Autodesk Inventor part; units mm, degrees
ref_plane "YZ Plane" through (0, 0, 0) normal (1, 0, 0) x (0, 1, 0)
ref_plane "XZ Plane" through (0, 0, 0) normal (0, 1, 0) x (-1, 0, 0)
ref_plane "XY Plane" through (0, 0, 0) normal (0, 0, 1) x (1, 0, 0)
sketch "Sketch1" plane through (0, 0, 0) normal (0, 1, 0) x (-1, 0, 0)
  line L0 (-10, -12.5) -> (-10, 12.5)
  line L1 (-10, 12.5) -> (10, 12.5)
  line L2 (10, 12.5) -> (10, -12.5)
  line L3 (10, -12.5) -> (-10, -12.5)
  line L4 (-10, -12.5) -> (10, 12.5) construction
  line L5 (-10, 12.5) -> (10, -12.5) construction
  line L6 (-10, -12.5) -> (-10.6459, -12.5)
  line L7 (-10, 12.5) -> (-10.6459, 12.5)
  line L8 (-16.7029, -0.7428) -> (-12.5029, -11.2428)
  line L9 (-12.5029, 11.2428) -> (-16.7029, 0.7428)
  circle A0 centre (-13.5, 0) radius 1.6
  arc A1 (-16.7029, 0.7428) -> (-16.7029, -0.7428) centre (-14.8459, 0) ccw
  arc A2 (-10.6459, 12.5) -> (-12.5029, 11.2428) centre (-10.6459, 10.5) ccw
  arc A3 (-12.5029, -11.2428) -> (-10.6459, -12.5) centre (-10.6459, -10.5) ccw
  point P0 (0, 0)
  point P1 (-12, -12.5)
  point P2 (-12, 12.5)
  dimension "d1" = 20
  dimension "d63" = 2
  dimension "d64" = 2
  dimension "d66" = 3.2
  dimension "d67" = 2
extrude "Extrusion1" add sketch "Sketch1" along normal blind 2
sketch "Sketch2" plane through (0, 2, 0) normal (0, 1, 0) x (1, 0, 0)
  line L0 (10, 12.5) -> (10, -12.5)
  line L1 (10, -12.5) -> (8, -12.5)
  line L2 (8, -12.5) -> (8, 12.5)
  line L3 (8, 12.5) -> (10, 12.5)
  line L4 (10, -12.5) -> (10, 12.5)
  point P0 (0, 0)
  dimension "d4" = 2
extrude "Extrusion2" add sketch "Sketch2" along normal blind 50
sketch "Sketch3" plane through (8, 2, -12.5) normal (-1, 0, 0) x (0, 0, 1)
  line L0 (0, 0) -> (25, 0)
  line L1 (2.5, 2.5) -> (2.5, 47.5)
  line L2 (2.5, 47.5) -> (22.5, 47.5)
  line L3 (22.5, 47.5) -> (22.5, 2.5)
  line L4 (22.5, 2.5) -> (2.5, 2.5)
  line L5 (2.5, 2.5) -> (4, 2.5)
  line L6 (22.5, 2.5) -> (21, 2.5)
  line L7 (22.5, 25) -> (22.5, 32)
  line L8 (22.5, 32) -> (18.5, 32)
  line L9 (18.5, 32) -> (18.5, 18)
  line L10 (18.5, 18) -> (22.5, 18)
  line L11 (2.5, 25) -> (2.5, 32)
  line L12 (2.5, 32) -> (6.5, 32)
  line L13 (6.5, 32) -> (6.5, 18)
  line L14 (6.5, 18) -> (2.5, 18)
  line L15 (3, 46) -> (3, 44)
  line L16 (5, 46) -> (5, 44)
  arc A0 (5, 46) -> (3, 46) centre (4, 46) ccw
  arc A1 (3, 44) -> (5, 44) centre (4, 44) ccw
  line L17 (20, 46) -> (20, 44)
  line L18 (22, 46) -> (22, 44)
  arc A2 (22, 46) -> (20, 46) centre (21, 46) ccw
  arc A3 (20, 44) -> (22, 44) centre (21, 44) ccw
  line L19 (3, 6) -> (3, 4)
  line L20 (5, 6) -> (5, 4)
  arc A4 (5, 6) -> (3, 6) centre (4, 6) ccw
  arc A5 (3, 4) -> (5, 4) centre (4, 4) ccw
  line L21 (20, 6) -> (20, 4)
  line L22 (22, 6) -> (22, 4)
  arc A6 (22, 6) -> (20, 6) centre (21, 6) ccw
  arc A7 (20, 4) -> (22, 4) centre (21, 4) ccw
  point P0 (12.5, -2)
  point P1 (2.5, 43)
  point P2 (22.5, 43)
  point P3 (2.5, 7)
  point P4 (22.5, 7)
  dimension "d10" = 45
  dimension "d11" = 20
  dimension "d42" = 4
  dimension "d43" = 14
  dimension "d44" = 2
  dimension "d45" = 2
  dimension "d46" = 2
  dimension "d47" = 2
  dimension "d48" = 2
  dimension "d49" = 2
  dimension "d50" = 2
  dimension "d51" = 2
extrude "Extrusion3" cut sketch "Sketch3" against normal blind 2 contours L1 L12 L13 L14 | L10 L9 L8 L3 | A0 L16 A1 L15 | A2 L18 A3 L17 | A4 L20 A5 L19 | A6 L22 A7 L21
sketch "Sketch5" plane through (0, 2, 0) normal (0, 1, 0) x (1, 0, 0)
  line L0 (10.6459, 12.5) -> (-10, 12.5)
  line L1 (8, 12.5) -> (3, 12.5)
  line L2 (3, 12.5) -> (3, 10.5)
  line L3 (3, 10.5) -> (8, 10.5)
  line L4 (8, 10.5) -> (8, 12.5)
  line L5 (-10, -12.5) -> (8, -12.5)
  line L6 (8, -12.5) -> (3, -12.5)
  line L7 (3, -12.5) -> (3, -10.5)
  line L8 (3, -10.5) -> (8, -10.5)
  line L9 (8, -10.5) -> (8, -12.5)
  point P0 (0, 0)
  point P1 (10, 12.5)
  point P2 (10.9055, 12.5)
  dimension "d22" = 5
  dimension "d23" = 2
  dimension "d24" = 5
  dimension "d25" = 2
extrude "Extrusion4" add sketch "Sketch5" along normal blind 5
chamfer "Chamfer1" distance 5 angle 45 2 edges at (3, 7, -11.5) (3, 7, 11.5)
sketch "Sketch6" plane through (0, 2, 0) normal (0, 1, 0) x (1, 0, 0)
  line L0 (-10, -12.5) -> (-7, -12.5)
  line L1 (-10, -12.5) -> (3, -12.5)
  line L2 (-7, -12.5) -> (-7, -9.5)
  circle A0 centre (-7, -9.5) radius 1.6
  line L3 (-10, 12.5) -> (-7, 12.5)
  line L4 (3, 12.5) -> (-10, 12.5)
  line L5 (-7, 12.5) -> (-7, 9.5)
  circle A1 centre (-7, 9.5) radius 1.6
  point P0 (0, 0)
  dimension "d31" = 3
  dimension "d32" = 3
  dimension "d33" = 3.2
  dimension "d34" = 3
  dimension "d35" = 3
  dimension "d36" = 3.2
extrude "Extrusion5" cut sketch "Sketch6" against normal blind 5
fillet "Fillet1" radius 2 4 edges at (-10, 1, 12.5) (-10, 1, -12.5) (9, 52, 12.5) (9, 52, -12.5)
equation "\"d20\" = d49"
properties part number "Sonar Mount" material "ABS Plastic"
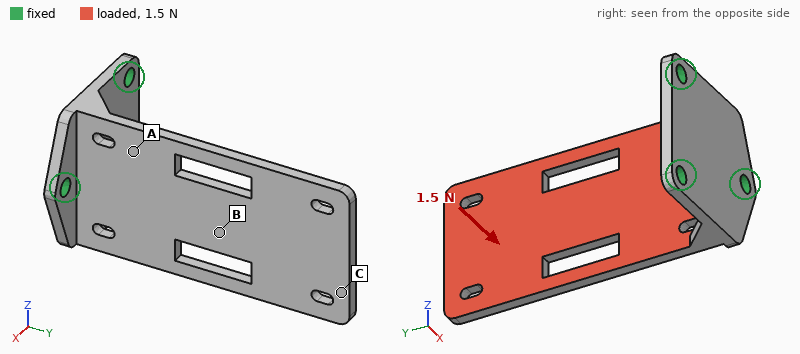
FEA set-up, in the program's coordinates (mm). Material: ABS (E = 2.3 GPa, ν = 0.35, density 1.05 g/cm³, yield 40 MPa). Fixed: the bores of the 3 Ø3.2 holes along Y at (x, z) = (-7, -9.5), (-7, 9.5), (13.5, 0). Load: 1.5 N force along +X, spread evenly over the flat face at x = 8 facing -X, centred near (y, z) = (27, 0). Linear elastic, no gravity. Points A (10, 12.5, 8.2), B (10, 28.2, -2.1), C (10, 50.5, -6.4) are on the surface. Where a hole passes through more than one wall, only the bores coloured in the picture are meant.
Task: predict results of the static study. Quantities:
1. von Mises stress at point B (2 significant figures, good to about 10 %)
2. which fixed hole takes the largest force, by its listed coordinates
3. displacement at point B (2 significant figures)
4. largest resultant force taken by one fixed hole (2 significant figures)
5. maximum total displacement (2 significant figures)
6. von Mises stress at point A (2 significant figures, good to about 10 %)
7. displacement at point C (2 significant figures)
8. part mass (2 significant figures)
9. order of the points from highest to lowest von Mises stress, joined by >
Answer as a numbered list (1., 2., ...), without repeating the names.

1. 0.81 MPa
2. (13.5, 0)
3. 0.26 mm
4. 2.6 N
5. 0.71 mm
6. 1.4 MPa
7. 0.68 mm
8. 3.6 g
9. A > B > C
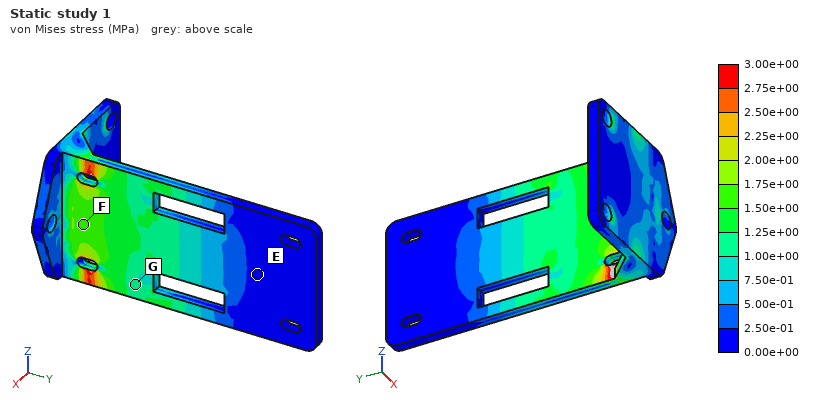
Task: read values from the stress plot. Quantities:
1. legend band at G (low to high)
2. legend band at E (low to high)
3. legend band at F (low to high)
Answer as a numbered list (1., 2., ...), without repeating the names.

1. 1.00e+00 to 1.25e+00 MPa
2. 0.00e+00 to 2.50e-01 MPa
3. 1.50e+00 to 1.75e+00 MPa
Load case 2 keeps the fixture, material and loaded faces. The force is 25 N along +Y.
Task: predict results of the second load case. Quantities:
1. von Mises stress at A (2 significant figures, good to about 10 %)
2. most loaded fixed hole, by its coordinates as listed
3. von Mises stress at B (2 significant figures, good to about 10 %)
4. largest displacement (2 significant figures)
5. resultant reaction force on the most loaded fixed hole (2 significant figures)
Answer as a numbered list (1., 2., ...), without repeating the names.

1. 0.90 MPa
2. (13.5, 0)
3. 0.73 MPa
4. 0.68 mm
5. 20 N
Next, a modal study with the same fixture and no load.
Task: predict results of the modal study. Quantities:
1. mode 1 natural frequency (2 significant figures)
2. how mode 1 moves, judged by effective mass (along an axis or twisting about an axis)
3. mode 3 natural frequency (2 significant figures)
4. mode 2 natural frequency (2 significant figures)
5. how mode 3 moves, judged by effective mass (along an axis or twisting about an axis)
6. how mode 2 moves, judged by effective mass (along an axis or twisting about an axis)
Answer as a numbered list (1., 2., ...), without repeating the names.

1. 190 Hz
2. along X
3. 790 Hz
4. 540 Hz
5. twisting about Y
6. along Z
